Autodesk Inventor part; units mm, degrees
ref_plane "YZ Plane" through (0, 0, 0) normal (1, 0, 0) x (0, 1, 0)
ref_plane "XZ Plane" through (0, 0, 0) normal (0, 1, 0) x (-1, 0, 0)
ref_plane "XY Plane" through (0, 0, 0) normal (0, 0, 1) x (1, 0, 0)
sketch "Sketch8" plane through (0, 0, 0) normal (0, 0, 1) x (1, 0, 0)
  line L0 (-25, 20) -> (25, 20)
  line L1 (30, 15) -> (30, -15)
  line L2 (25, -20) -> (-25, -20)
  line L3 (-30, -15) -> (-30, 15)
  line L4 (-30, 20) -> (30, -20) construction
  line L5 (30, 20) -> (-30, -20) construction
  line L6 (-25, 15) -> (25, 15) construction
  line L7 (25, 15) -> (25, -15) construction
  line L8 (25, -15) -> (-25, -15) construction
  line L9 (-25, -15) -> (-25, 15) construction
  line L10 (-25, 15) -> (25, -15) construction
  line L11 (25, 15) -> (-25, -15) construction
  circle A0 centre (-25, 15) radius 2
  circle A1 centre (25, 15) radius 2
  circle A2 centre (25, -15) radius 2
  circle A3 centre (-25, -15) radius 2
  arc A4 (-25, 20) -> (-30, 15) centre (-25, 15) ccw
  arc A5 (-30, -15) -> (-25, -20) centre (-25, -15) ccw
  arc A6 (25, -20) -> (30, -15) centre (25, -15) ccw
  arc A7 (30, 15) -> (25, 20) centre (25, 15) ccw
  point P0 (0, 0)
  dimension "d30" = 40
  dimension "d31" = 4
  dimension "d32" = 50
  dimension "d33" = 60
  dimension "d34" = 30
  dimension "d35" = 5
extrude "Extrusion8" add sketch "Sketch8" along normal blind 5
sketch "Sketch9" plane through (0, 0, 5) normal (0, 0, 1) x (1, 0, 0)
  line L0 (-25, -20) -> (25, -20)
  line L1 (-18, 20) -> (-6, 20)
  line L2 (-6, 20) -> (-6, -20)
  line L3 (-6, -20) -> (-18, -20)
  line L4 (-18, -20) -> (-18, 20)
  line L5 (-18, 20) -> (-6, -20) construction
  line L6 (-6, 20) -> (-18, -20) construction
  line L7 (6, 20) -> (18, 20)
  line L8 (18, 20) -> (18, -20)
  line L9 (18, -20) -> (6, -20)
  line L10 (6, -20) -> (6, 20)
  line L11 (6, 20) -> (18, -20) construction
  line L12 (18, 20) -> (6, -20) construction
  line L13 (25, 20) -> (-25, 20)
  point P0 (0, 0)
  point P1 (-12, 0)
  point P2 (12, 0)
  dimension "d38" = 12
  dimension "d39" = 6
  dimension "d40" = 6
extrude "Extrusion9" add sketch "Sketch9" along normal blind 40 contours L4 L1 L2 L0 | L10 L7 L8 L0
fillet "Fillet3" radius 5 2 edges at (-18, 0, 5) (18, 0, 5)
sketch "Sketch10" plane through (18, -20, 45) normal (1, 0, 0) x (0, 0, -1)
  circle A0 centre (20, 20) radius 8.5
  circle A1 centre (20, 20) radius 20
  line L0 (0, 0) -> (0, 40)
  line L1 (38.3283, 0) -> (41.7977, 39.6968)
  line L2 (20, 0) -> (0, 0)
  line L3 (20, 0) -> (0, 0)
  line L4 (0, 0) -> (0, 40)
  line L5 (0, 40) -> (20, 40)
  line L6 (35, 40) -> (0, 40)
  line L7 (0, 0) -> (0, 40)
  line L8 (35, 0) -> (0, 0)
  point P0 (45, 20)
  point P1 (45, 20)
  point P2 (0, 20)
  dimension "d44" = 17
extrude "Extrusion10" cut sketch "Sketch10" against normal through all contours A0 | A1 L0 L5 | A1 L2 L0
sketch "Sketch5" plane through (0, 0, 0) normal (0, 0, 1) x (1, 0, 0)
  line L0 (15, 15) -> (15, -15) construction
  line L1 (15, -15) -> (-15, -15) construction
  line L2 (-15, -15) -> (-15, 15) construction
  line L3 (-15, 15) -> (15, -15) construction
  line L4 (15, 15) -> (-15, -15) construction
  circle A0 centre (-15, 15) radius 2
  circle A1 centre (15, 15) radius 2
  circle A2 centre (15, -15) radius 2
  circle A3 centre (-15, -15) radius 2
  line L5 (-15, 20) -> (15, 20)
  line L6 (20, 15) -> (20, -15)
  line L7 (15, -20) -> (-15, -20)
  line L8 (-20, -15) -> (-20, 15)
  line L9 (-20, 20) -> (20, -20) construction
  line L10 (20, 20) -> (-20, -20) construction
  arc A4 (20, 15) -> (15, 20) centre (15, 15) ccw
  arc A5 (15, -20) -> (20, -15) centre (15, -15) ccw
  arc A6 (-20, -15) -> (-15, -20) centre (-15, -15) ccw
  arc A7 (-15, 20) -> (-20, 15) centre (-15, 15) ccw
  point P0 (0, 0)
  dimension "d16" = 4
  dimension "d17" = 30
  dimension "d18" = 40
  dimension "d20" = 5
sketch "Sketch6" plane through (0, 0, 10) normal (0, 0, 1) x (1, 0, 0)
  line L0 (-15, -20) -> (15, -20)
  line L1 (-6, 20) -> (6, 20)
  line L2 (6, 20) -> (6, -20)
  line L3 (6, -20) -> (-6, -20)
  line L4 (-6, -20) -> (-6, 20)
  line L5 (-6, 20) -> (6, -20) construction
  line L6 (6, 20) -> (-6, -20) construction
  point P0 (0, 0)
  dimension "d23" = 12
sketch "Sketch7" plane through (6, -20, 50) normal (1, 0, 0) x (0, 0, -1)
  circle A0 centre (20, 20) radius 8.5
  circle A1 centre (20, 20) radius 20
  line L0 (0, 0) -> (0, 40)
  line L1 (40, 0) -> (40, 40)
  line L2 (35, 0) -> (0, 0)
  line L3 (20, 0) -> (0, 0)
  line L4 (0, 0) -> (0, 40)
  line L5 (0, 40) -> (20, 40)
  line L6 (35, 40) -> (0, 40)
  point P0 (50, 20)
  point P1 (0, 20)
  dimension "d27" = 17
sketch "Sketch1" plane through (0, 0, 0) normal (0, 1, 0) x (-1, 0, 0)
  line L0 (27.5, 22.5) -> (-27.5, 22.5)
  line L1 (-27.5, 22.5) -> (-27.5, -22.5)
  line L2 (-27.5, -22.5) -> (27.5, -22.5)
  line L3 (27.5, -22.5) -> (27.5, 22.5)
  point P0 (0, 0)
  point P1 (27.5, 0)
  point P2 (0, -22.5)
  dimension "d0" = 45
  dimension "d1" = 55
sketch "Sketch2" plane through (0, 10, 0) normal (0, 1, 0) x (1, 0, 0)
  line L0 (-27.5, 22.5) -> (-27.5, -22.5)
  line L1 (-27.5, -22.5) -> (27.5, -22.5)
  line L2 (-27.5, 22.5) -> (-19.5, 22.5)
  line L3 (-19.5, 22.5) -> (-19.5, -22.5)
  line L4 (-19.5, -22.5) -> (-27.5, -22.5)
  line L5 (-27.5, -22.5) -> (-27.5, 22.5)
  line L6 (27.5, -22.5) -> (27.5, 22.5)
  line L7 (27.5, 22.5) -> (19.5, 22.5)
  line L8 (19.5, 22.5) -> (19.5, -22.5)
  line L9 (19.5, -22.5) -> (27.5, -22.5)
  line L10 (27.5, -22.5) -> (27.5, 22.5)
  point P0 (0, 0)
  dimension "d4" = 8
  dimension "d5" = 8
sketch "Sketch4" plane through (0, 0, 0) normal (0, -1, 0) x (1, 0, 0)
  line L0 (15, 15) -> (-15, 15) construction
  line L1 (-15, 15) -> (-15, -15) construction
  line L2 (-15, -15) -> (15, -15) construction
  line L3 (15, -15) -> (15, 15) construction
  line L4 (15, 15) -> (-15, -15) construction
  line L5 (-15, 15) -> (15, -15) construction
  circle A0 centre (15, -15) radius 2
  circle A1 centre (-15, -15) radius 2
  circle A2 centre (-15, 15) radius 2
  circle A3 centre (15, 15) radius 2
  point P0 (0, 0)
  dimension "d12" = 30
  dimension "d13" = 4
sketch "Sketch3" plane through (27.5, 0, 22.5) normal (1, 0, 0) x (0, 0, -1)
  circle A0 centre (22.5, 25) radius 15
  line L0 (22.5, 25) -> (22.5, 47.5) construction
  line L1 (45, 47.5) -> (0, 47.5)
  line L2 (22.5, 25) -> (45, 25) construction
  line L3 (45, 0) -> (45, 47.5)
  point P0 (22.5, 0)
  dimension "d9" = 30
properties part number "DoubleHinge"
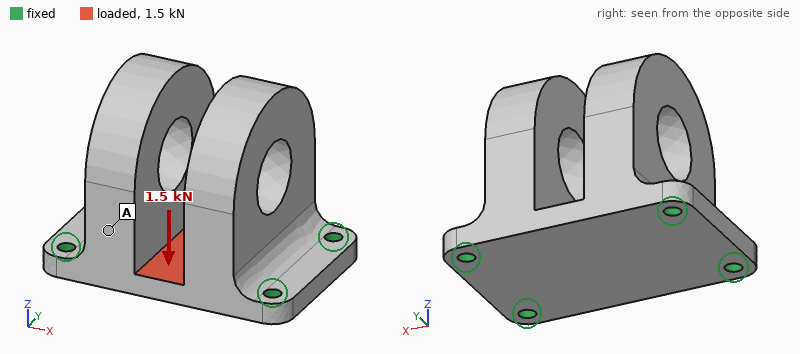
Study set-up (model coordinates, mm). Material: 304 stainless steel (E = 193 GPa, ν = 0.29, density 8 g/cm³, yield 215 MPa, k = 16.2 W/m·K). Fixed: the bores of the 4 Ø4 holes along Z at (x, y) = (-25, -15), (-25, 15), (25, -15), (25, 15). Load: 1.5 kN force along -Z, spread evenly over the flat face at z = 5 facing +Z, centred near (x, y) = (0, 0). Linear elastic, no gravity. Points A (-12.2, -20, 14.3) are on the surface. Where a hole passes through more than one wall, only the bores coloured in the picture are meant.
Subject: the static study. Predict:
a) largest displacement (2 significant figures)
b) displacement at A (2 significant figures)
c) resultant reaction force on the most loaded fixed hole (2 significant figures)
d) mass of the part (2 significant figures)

29 µm
10 µm
380 N
330 g
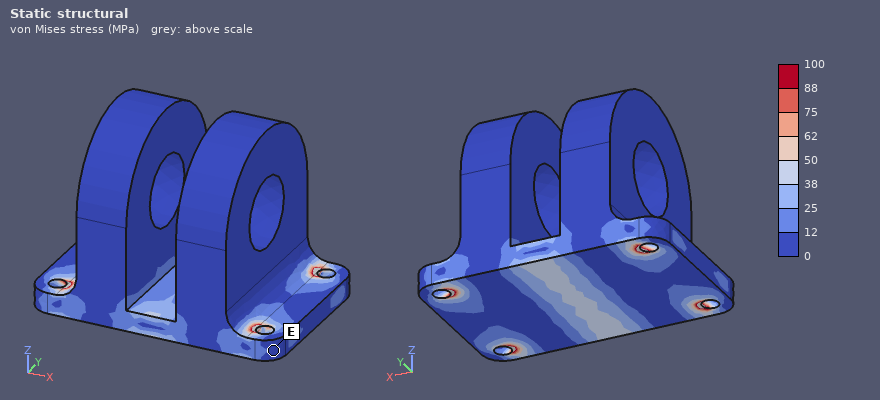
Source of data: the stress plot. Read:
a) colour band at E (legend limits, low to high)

0 to 12 MPa
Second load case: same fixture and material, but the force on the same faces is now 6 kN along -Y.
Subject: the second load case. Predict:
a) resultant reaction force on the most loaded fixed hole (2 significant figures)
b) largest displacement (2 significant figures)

1.9 kN
5.7 µm
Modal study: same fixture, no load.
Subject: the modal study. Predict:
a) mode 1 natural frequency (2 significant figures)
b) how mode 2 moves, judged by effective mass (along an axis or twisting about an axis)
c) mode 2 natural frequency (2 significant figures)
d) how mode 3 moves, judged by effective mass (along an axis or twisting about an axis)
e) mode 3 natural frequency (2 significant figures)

2400 Hz
along X
4900 Hz
along Y
5300 Hz
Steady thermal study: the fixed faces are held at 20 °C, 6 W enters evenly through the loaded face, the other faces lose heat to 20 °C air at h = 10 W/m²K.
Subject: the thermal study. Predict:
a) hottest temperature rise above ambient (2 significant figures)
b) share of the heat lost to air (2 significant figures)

17 K
17 %
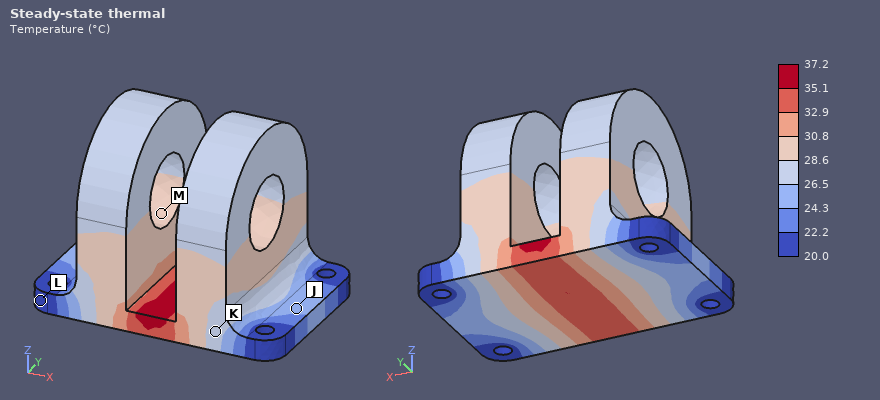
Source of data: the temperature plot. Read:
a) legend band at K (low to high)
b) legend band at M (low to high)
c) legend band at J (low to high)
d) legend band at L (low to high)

26.5 to 28.6 °C
28.6 to 30.8 °C
24.3 to 26.5 °C
20.0 to 22.2 °C
